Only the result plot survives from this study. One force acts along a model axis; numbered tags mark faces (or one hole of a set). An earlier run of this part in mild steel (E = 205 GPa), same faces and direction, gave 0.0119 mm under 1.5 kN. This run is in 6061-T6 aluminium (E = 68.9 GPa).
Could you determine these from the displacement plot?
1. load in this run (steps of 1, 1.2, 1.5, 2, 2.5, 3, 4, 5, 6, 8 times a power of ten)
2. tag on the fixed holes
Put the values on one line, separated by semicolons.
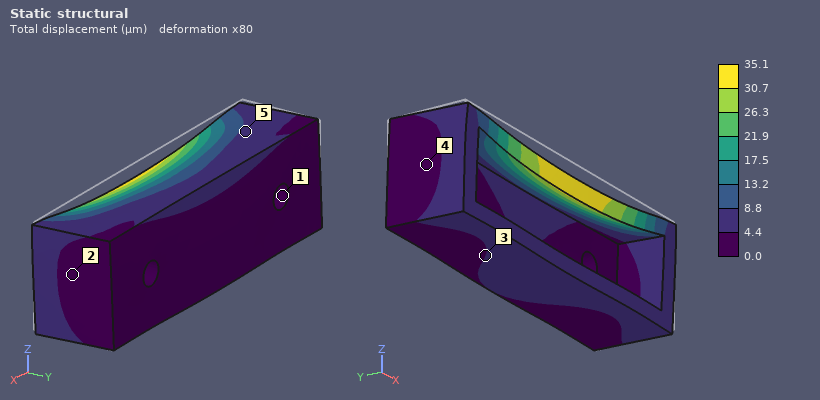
1.5 kN; 1
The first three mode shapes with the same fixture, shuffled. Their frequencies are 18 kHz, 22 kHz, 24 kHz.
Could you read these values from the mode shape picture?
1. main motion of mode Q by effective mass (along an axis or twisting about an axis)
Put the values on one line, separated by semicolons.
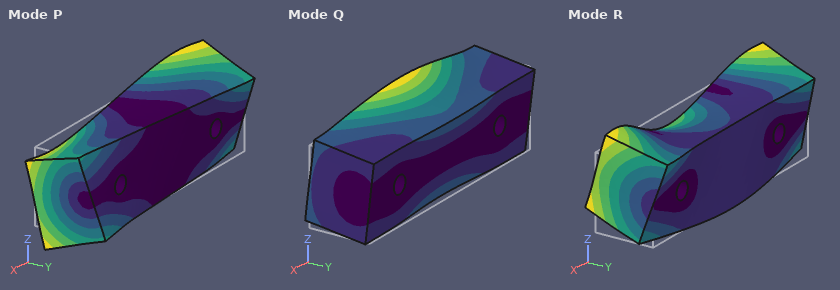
along Z
